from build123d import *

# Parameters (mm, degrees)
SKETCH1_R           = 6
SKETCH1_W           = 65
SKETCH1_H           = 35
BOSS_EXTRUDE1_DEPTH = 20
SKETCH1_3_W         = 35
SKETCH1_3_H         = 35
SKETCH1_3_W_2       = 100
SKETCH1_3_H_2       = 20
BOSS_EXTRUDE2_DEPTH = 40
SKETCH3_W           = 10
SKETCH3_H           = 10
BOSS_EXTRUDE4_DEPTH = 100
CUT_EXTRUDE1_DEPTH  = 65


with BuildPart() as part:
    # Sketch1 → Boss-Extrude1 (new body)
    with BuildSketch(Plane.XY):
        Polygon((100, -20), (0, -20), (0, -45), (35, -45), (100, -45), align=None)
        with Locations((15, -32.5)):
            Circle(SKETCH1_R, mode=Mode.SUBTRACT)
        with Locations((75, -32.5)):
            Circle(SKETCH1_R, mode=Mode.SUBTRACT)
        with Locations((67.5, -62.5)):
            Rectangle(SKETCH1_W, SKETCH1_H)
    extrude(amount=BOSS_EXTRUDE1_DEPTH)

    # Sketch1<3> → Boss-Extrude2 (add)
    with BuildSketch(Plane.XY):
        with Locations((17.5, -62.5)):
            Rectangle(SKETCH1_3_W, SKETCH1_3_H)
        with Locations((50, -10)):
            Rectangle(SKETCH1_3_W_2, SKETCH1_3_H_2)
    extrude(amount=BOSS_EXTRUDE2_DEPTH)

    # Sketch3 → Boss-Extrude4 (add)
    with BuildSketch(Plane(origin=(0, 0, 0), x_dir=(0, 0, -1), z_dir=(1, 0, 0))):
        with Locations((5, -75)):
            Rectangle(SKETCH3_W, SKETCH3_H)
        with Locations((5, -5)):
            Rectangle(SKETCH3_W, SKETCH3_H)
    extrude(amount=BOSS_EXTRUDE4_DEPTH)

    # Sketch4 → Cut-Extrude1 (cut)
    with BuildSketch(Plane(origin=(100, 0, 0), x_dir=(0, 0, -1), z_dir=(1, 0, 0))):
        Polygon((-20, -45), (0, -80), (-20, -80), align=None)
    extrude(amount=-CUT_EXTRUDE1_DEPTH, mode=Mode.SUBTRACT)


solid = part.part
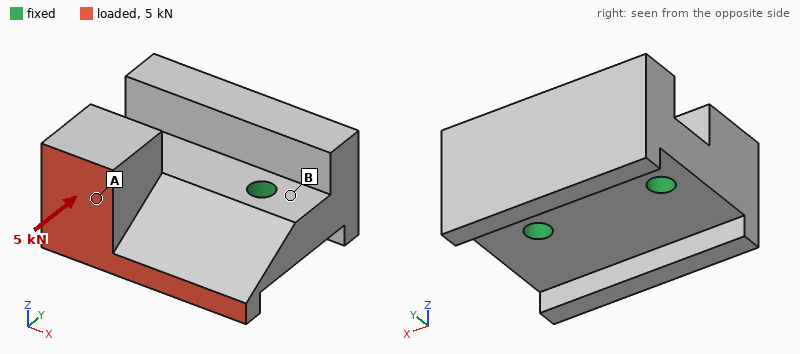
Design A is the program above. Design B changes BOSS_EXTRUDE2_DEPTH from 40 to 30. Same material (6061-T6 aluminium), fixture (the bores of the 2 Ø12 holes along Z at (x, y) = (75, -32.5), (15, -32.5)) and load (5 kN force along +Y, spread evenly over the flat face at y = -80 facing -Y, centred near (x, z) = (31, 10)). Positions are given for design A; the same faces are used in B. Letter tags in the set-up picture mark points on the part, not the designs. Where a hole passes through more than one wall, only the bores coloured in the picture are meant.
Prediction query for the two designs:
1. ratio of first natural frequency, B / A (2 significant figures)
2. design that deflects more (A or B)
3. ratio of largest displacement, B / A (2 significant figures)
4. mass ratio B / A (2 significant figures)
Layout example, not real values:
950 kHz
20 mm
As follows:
1.2
B
1.2
0.85
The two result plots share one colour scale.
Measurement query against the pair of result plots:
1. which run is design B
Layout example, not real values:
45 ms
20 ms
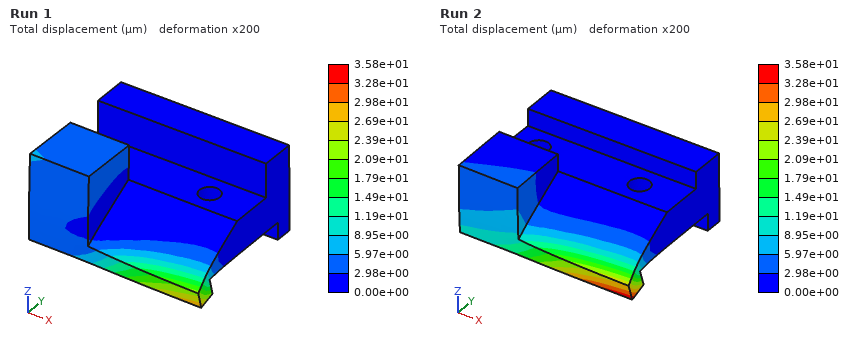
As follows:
Run 2
